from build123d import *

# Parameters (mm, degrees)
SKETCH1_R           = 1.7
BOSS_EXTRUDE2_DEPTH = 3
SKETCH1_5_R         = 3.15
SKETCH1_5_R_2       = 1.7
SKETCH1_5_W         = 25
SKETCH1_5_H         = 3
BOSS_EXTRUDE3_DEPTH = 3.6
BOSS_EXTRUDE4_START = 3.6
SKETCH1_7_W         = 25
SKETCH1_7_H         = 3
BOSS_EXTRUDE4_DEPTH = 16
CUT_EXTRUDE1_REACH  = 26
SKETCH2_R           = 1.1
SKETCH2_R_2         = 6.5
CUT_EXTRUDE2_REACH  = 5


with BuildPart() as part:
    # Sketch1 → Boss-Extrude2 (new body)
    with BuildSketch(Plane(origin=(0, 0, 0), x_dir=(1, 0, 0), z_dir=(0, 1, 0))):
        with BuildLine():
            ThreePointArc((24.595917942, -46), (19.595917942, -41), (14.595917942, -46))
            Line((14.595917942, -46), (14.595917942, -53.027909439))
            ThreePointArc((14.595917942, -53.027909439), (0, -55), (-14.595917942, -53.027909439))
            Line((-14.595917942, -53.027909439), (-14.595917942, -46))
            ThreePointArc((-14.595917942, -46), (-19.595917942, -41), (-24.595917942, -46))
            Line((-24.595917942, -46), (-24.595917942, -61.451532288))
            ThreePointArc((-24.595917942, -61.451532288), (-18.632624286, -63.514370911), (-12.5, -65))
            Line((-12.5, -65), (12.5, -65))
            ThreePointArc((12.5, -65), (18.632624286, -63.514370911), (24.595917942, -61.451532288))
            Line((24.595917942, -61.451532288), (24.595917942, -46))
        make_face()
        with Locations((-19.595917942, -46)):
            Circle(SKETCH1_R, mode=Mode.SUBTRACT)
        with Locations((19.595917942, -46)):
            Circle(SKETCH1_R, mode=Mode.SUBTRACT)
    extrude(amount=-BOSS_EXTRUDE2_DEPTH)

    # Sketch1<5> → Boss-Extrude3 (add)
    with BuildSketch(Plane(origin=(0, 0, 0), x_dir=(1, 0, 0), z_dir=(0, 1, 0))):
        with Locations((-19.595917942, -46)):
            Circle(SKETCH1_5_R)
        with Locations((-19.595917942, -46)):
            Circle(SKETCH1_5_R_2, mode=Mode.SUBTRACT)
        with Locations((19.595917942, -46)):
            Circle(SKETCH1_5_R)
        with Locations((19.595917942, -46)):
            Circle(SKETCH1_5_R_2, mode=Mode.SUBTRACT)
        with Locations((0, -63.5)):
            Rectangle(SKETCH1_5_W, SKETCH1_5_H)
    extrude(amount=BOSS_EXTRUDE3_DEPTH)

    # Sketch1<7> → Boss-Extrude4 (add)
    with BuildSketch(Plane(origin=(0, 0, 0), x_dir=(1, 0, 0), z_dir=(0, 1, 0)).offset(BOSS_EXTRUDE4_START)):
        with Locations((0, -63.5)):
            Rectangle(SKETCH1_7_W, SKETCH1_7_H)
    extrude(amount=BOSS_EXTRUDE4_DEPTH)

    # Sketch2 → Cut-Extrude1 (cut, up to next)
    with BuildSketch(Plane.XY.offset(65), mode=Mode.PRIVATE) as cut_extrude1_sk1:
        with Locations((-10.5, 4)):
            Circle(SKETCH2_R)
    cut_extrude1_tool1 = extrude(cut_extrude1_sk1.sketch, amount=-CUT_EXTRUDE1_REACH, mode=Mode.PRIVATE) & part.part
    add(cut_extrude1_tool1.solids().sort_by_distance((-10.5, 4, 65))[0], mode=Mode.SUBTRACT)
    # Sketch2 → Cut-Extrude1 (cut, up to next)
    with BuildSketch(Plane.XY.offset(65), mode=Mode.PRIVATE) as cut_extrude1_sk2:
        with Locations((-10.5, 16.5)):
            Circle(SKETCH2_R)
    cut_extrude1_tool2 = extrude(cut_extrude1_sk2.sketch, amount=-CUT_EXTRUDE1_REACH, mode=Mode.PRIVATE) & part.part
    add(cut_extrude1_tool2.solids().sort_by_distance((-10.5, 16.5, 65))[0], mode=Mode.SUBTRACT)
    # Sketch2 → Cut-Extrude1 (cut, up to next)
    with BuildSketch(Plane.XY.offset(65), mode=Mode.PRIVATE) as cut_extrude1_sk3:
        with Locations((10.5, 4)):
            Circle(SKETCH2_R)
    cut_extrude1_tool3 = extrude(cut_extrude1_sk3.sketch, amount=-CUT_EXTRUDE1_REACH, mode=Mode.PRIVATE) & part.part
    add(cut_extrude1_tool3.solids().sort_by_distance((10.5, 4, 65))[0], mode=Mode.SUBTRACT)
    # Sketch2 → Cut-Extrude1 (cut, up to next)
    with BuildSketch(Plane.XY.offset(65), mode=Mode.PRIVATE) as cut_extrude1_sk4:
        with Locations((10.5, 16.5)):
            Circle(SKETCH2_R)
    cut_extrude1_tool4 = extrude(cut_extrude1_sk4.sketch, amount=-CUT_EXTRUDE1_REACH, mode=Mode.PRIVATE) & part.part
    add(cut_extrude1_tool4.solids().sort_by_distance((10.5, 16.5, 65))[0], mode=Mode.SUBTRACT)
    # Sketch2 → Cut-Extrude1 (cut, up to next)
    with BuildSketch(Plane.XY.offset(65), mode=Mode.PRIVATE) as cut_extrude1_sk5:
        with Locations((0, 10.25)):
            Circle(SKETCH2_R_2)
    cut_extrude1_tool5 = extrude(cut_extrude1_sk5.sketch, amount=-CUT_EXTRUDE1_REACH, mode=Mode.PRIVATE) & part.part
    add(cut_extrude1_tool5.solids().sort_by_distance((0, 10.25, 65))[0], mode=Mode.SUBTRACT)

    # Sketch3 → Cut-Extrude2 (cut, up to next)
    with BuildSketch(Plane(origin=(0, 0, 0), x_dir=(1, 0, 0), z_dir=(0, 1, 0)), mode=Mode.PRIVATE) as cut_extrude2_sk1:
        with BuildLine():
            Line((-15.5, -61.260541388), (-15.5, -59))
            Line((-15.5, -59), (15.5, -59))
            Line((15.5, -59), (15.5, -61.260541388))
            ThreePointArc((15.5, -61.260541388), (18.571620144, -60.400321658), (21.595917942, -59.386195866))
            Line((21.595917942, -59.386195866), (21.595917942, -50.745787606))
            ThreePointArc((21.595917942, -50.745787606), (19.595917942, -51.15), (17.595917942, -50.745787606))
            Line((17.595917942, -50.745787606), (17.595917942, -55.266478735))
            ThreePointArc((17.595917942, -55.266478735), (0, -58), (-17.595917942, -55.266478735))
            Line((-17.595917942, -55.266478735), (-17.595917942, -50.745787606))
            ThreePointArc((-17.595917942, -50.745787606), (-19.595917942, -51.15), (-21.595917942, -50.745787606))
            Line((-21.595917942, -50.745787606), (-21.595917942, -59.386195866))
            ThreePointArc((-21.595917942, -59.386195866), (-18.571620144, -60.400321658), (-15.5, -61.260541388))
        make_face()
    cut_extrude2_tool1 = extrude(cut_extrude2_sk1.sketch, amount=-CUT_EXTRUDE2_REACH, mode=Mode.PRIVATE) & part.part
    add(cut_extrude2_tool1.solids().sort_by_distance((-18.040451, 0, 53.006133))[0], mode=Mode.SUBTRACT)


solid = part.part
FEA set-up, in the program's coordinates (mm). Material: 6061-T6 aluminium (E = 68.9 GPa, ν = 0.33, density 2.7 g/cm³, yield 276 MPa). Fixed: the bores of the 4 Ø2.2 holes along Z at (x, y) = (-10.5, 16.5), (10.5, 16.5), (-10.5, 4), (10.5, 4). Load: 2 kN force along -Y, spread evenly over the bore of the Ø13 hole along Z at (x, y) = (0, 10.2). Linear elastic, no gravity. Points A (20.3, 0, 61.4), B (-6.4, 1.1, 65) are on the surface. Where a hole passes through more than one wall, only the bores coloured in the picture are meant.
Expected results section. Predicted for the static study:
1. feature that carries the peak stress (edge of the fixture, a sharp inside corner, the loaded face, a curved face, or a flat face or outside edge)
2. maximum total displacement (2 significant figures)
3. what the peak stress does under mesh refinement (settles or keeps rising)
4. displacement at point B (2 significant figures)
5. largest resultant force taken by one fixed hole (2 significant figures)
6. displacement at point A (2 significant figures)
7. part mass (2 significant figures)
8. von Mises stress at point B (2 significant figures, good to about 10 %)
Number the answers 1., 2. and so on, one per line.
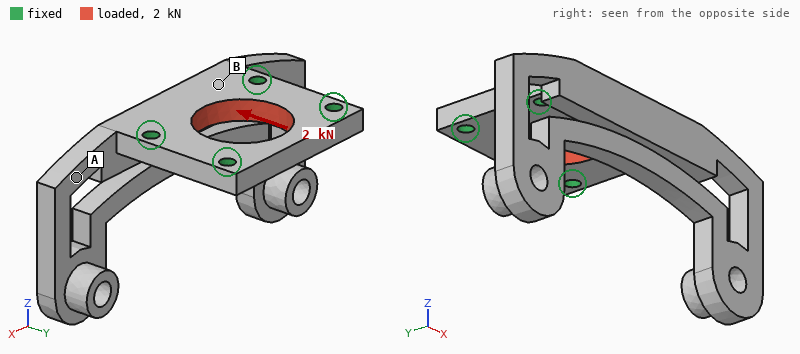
1. edge of the fixture
2. 13 µm
3. keeps rising
4. 2.8 µm
5. 570 N
6. 4.2 µm
7. 7.8 g
8. 18 MPa
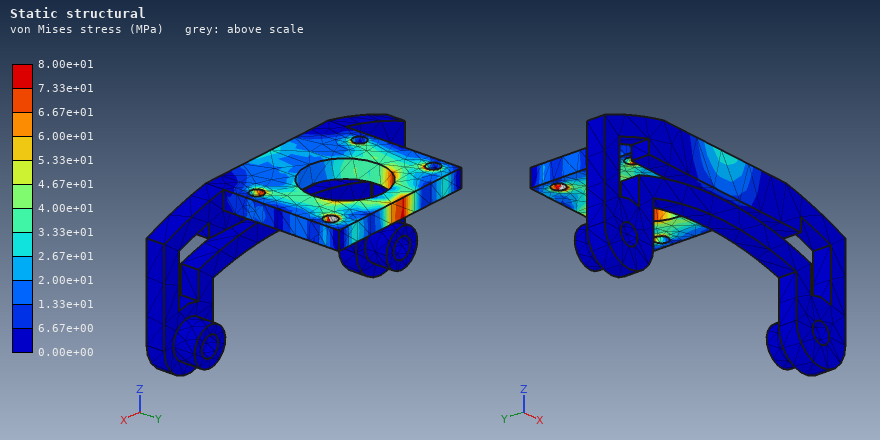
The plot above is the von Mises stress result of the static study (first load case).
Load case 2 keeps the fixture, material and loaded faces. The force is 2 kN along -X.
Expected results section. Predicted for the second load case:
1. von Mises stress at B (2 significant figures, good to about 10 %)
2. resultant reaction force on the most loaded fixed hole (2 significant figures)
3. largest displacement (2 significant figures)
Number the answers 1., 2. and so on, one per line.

1. 9.8 MPa
2. 510 N
3. 3.0 µm
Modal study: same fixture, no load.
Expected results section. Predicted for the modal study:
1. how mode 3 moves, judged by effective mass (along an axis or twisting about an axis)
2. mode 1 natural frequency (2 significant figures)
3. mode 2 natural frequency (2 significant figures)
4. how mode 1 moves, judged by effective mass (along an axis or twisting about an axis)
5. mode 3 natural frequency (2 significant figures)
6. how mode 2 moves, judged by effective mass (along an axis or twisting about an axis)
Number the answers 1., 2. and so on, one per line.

1. along X
2. 1500 Hz
3. 2000 Hz
4. along Y
5. 2700 Hz
6. twisting about Z
